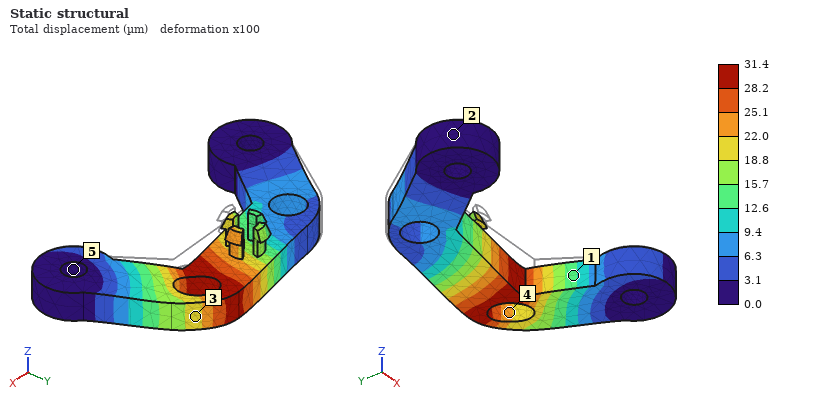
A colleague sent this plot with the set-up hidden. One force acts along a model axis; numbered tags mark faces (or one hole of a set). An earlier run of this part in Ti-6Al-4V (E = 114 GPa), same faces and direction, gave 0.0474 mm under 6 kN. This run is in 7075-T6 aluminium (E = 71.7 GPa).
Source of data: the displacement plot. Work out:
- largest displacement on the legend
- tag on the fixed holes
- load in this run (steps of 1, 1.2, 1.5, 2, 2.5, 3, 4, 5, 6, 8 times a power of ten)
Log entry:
31.4 µm
5
2.5 kN
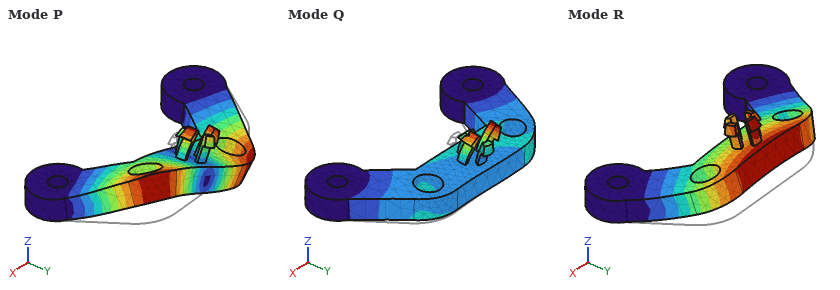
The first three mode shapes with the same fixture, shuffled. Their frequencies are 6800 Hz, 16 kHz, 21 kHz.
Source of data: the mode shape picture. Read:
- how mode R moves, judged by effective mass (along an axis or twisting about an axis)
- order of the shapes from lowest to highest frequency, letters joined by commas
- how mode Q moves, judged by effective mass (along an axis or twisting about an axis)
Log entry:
along Z
R, P, Q
along X
